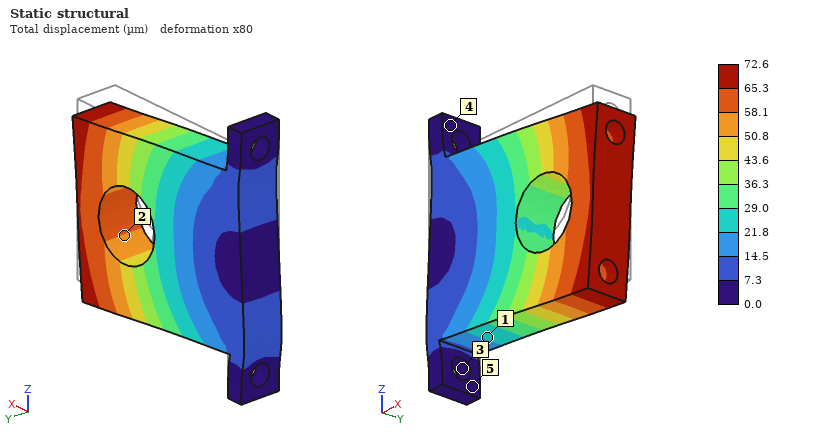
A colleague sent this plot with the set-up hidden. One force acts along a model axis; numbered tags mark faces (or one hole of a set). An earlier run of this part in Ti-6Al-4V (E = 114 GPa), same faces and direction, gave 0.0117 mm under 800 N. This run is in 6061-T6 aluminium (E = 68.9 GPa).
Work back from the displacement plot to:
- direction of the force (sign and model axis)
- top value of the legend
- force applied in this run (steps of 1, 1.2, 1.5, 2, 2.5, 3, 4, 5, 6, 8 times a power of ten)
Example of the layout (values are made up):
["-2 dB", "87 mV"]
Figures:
["-Z", "72.6 µm", "3 kN"]
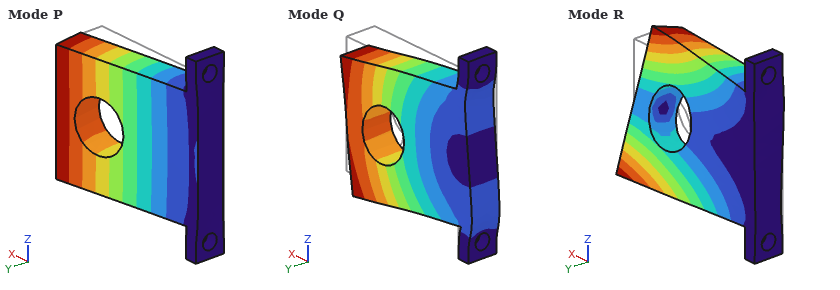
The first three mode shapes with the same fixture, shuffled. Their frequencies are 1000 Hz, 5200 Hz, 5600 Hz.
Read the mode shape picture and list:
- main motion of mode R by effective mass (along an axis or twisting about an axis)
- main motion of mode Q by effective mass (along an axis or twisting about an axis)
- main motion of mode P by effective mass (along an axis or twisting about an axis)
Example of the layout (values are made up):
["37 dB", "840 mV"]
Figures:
["twisting about X", "along Z", "along Y"]
